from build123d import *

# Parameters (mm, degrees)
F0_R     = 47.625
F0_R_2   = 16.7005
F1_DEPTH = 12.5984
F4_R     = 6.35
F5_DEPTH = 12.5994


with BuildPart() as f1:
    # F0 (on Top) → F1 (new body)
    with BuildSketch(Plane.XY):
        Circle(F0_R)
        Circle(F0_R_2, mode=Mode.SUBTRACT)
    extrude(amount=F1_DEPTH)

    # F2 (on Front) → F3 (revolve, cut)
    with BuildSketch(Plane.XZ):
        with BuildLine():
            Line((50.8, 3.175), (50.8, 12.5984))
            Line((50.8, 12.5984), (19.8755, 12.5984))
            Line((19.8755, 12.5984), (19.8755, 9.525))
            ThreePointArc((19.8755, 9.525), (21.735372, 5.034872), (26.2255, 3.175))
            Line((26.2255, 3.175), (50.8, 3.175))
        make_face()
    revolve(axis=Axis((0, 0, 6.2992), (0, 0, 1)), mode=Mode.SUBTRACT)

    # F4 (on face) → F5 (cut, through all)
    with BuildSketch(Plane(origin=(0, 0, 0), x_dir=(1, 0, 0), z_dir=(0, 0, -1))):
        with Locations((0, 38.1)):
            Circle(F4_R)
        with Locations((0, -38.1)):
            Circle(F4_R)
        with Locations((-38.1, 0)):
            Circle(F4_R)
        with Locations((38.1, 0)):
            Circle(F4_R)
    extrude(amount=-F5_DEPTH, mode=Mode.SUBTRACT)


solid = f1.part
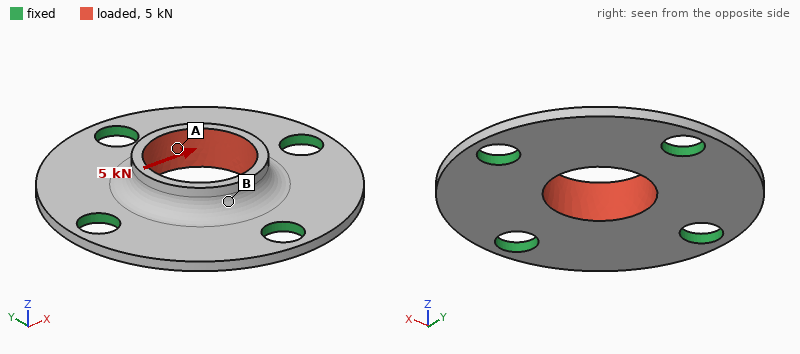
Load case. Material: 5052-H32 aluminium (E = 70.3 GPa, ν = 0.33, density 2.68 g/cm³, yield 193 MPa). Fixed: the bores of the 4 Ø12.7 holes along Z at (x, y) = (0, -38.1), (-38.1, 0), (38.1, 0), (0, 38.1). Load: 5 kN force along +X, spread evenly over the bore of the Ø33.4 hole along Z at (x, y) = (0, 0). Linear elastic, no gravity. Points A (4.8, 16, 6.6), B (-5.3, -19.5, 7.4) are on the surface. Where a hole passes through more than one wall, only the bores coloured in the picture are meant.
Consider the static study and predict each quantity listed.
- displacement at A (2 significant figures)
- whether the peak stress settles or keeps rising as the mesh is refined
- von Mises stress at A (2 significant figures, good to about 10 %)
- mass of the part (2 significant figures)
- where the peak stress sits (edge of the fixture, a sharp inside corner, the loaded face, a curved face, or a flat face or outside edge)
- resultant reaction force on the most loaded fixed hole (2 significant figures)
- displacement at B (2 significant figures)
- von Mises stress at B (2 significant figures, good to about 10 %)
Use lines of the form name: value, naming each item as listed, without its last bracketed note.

displacement at A: 8.7 µm
whether the peak stress settles or keeps rising as the mesh is refined: keeps rising
von Mises stress at A: 19 MPa
mass of the part: 61 g
where the peak stress sits: edge of the fixture
resultant reaction force on the most loaded fixed hole: 1.6 kN
displacement at B: 8.3 µm
von Mises stress at B: 8.0 MPa
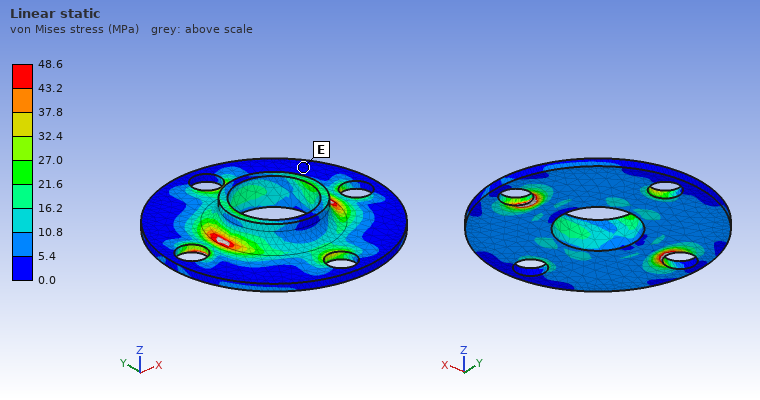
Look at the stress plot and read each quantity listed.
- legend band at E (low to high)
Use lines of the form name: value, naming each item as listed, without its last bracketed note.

legend band at E: 0.0 to 5.4 MPa
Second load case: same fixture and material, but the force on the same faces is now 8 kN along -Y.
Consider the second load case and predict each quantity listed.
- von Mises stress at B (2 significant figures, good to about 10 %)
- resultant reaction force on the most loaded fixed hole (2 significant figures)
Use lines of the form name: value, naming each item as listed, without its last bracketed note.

von Mises stress at B: 27 MPa
resultant reaction force on the most loaded fixed hole: 2.5 kN
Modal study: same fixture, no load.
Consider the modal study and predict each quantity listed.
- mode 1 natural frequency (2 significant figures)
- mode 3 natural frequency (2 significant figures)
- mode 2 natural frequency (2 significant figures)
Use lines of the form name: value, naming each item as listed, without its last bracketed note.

mode 1 natural frequency: 6400 Hz
mode 3 natural frequency: 6600 Hz
mode 2 natural frequency: 6600 Hz
